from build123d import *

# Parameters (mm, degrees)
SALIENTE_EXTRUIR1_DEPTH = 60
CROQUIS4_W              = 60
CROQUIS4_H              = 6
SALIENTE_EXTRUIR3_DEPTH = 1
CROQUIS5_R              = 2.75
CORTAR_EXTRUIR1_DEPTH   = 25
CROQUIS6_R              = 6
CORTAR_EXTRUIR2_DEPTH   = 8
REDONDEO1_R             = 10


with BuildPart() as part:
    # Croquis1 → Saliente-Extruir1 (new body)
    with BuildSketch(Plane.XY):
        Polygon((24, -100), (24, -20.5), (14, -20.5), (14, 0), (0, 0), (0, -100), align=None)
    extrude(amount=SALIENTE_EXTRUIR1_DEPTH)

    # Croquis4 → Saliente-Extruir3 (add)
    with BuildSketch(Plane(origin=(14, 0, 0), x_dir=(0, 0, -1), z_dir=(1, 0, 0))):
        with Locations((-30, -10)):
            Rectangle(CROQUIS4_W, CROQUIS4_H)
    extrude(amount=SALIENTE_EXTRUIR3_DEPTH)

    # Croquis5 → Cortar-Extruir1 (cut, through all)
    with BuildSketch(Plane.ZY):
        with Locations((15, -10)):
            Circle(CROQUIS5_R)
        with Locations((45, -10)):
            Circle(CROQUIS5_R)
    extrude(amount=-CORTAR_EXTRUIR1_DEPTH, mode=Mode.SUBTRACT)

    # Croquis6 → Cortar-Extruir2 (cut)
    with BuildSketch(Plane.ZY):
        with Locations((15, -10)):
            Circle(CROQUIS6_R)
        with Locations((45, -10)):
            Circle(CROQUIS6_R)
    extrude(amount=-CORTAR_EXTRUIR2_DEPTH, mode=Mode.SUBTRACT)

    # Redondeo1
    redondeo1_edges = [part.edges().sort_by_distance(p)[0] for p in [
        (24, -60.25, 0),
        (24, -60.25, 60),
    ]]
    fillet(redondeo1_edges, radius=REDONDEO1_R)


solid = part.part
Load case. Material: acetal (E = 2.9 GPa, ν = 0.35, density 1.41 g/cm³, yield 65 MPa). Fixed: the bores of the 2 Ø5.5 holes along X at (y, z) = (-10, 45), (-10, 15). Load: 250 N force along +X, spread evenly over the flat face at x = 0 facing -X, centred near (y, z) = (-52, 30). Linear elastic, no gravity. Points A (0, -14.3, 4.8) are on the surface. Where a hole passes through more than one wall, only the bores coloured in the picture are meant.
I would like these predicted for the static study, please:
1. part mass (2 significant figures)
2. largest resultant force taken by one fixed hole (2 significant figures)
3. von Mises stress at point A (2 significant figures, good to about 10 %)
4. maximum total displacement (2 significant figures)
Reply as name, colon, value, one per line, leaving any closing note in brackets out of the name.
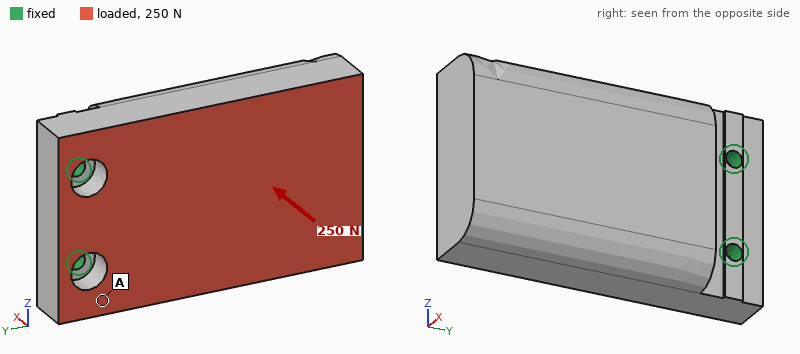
part mass: 180 g
largest resultant force taken by one fixed hole: 130 N
von Mises stress at point A: 5.2 MPa
maximum total displacement: 1.2 mm
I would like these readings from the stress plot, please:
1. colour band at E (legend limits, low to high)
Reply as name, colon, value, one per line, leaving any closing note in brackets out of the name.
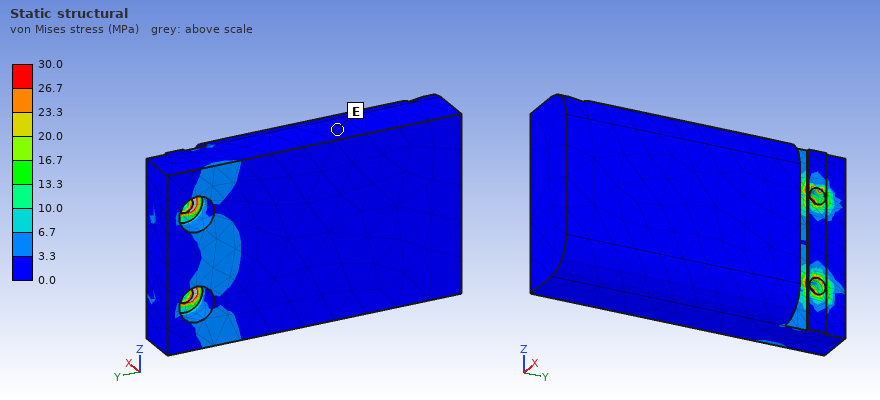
colour band at E: 0.0 to 3.3 MPa
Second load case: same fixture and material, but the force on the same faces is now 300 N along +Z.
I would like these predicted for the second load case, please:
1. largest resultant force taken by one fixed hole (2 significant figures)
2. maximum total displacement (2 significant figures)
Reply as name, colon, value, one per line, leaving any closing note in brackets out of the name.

largest resultant force taken by one fixed hole: 420 N
maximum total displacement: 0.12 mm
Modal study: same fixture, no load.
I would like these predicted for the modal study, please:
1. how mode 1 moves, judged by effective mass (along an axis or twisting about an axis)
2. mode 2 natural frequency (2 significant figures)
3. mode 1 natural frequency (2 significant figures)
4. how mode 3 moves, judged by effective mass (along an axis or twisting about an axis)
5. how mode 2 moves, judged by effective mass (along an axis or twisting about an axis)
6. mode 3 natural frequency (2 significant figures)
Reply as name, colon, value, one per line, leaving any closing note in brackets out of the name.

how mode 1 moves, judged by effective mass: along X
mode 2 natural frequency: 730 Hz
mode 1 natural frequency: 200 Hz
how mode 3 moves, judged by effective mass: twisting about Y
how mode 2 moves, judged by effective mass: along Z
mode 3 natural frequency: 1200 Hz
